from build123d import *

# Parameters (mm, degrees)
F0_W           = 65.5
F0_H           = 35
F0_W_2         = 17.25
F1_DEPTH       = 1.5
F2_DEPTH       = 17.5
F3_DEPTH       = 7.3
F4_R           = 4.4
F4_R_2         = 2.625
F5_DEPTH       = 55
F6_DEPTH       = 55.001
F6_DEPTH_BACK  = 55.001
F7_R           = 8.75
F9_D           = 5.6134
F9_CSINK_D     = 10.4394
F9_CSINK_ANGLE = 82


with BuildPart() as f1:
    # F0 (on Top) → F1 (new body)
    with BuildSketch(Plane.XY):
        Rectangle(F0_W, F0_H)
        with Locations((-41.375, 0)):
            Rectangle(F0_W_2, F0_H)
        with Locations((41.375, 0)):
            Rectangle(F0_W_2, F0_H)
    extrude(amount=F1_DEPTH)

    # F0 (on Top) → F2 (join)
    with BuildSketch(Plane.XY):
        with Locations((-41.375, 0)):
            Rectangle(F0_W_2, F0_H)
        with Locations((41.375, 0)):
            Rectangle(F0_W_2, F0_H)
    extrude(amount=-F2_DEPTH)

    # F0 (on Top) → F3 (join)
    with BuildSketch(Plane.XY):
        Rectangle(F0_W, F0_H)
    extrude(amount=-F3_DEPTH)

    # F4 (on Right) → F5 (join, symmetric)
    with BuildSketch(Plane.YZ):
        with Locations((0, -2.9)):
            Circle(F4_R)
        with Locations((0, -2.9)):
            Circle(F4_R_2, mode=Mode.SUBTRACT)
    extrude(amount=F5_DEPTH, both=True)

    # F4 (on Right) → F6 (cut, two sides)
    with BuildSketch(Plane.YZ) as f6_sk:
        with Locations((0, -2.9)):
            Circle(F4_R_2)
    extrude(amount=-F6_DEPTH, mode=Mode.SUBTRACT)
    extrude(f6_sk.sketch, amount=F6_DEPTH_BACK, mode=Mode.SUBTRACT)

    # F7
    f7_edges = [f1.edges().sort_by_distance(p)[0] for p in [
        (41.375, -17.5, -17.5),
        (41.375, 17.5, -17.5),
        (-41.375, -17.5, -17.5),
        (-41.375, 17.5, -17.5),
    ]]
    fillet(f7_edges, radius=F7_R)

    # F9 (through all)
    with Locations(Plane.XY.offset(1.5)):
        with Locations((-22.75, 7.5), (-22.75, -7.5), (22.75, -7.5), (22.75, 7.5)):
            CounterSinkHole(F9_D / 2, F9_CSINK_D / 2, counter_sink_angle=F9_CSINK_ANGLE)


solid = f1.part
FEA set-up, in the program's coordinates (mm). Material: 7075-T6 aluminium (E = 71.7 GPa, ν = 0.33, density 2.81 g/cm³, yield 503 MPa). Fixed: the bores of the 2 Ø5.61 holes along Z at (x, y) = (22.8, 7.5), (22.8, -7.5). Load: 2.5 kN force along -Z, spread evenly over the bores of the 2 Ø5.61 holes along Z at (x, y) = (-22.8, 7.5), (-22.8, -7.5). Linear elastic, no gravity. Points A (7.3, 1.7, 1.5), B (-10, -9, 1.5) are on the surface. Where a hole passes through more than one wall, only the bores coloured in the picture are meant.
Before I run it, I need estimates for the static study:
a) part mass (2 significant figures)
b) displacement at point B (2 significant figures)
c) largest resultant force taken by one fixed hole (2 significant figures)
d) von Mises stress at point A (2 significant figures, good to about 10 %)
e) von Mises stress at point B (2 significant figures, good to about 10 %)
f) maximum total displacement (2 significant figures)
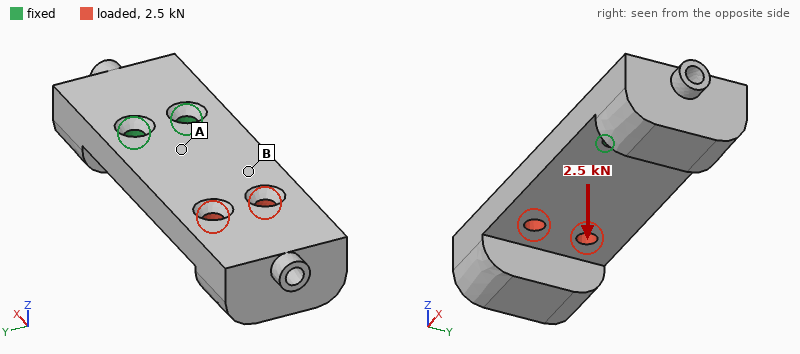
110 g
0.41 mm
1.3 kN
150 MPa
72 MPa
1.3 mm
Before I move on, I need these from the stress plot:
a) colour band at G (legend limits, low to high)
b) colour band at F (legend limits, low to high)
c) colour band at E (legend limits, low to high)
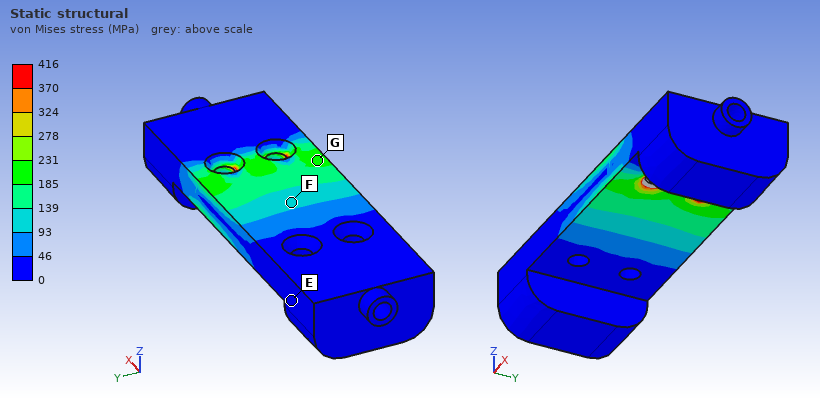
185 to 231 MPa
93 to 139 MPa
0 to 46 MPa
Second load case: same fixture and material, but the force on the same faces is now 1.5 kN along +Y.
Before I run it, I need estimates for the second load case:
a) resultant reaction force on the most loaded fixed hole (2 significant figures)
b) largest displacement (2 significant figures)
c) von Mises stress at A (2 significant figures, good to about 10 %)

3.5 kN
81 µm
21 MPa
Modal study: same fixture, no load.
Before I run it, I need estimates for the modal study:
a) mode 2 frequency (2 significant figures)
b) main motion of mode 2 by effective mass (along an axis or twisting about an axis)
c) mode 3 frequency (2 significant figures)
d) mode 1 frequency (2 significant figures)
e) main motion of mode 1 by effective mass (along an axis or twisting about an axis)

2900 Hz
along Y
4100 Hz
960 Hz
along Z
